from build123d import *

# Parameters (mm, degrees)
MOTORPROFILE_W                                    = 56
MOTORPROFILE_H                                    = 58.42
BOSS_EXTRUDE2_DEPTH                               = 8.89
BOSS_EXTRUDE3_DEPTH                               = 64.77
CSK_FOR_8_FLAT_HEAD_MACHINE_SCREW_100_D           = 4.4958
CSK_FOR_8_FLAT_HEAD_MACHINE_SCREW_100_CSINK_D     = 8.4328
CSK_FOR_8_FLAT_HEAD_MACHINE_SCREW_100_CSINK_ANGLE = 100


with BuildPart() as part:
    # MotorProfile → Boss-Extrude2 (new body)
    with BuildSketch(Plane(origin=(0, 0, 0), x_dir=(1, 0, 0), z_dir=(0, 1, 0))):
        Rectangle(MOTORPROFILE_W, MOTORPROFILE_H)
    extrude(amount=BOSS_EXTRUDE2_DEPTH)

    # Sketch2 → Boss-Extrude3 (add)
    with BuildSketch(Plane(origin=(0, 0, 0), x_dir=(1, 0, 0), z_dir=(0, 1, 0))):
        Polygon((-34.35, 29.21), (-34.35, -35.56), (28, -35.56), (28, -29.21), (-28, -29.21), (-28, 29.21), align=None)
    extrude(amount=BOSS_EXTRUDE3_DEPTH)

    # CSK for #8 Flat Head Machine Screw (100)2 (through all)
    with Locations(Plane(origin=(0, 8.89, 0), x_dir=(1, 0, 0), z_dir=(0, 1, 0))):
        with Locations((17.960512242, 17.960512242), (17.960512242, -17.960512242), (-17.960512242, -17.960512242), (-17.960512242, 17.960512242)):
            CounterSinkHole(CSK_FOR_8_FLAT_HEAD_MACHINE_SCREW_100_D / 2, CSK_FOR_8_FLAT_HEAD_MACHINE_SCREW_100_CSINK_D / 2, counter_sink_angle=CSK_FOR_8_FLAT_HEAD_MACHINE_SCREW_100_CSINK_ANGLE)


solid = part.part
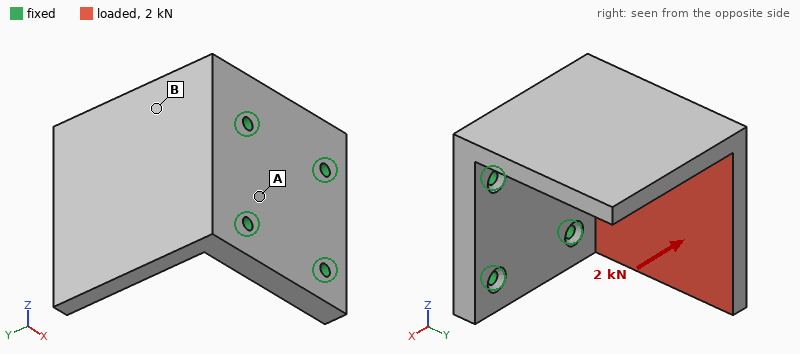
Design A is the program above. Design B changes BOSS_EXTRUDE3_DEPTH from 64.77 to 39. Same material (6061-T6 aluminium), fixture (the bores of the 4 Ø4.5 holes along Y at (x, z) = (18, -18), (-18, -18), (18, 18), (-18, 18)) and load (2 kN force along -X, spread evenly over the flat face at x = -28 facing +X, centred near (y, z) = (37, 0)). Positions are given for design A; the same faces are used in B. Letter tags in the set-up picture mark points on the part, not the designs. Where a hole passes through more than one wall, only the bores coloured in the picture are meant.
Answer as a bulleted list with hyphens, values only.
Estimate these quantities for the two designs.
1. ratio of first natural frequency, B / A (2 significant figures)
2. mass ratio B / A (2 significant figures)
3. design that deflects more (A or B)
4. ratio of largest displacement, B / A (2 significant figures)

- 2.2
- 0.75
- A
- 0.39
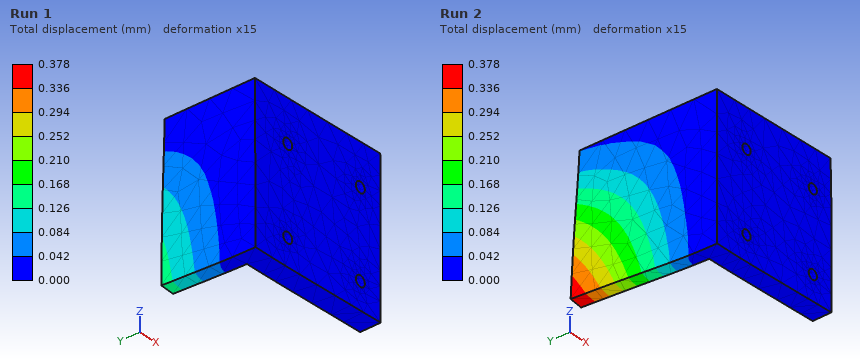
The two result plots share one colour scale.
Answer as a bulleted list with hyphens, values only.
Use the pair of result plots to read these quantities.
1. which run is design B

- Run 1
